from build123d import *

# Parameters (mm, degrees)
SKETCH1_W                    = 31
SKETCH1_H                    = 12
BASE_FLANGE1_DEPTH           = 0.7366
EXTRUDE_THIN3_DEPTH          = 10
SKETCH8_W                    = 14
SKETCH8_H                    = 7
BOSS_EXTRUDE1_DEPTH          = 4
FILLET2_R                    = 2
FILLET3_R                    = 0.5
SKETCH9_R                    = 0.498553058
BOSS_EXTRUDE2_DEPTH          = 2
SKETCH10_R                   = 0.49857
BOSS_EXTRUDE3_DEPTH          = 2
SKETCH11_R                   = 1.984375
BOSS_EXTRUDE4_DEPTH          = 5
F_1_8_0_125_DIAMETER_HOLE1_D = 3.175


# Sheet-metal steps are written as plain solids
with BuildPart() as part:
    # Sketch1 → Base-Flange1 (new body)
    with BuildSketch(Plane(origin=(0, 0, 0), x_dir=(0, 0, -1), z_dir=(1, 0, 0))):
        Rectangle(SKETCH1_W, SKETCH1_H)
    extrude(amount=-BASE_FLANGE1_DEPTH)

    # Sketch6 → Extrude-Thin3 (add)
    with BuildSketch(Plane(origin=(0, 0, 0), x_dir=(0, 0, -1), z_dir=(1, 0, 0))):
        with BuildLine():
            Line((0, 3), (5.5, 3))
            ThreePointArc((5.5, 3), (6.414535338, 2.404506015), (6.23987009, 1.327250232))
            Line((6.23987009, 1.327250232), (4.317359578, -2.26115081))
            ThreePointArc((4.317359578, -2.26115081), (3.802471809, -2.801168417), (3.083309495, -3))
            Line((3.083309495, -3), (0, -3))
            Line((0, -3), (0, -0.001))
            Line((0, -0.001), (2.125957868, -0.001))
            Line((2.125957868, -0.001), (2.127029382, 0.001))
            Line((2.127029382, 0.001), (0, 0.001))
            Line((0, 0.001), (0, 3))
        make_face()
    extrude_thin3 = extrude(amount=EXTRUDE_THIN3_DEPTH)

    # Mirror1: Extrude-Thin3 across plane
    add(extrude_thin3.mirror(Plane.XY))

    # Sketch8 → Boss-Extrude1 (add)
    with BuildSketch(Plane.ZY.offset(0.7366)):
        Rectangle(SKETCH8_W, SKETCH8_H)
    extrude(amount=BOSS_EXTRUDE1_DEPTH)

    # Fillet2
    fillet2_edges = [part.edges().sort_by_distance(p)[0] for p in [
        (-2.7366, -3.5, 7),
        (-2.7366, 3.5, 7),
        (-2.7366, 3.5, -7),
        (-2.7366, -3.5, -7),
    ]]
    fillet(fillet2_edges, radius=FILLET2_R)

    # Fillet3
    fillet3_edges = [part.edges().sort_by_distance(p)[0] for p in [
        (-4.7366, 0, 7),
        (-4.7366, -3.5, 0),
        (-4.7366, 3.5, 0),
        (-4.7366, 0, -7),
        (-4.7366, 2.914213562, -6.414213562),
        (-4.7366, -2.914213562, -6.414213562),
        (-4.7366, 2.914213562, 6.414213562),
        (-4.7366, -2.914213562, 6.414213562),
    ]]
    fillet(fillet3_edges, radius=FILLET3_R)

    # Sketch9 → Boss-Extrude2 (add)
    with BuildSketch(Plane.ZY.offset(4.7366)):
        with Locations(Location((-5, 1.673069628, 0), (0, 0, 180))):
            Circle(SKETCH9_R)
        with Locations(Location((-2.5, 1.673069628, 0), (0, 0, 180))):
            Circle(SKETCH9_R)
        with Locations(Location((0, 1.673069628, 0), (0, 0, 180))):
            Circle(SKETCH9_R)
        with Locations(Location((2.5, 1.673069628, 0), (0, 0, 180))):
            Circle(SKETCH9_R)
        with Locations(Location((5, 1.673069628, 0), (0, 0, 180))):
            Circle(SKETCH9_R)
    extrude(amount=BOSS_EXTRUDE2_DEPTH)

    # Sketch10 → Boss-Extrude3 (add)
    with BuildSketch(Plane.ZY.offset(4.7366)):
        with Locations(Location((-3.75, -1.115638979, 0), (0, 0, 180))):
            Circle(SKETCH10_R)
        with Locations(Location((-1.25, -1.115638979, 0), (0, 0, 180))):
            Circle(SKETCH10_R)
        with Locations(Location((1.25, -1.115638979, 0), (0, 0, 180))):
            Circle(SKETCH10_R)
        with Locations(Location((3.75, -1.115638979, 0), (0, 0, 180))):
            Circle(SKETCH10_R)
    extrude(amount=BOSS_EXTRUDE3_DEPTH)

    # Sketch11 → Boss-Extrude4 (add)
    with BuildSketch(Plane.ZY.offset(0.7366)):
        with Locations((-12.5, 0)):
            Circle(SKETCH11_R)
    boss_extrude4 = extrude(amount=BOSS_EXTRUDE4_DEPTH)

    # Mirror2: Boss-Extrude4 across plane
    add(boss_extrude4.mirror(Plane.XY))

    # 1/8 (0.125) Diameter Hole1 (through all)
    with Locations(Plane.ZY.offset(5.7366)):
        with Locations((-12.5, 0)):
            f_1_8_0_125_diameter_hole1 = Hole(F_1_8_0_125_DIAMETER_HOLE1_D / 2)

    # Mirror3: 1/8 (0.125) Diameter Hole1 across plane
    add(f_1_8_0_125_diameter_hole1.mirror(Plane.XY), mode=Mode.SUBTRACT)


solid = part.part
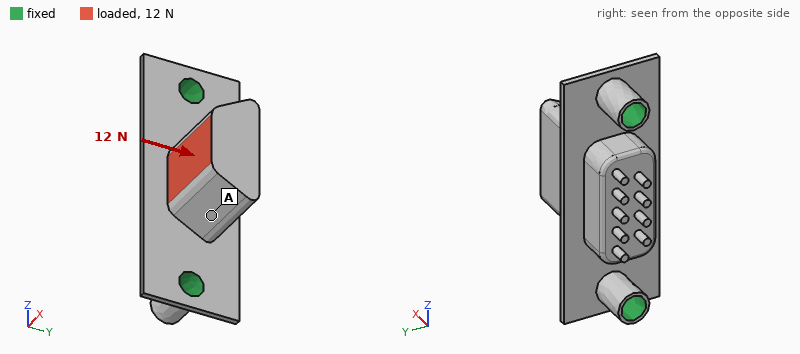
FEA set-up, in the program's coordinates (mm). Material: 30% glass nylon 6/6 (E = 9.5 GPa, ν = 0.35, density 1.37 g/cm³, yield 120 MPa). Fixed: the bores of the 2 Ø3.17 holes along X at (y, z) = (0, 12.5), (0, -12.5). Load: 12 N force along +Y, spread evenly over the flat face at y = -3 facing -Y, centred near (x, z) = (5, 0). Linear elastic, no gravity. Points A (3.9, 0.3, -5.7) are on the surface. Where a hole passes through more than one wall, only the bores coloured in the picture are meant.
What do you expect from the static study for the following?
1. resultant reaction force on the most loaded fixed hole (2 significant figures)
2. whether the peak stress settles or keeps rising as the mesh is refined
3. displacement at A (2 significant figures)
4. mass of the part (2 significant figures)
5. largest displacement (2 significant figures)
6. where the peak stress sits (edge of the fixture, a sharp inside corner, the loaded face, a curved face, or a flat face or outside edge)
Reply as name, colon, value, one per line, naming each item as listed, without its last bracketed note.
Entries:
resultant reaction force on the most loaded fixed hole: 6.1 N
whether the peak stress settles or keeps rising as the mesh is refined: keeps rising
displacement at A: 0.073 mm
mass of the part: 1.8 g
largest displacement: 0.18 mm
where the peak stress sits: edge of the fixture
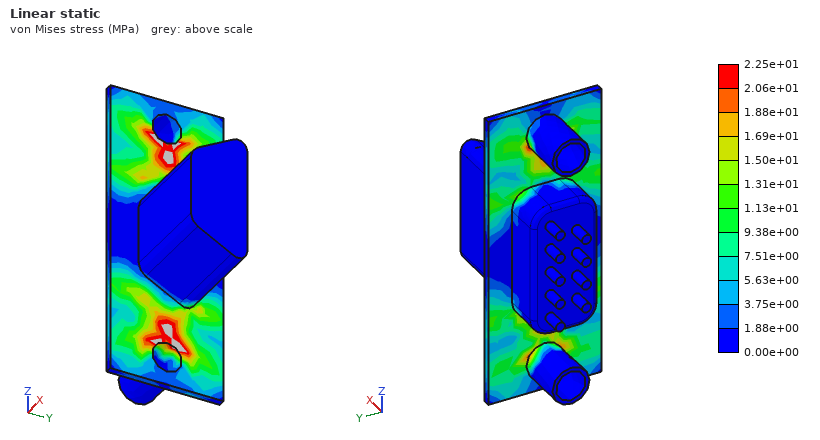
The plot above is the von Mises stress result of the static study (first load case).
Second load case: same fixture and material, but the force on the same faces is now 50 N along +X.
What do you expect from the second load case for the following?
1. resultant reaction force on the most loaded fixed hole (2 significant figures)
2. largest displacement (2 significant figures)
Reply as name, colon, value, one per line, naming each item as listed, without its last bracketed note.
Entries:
resultant reaction force on the most loaded fixed hole: 27 N
largest displacement: 0.45 mm
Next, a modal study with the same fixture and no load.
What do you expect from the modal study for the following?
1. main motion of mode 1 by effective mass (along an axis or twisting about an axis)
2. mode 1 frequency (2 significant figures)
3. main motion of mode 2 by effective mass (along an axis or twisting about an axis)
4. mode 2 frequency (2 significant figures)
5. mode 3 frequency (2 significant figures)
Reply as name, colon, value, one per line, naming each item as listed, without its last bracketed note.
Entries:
main motion of mode 1 by effective mass: along Y
mode 1 frequency: 1500 Hz
main motion of mode 2 by effective mass: along X
mode 2 frequency: 3100 Hz
mode 3 frequency: 4600 Hz
